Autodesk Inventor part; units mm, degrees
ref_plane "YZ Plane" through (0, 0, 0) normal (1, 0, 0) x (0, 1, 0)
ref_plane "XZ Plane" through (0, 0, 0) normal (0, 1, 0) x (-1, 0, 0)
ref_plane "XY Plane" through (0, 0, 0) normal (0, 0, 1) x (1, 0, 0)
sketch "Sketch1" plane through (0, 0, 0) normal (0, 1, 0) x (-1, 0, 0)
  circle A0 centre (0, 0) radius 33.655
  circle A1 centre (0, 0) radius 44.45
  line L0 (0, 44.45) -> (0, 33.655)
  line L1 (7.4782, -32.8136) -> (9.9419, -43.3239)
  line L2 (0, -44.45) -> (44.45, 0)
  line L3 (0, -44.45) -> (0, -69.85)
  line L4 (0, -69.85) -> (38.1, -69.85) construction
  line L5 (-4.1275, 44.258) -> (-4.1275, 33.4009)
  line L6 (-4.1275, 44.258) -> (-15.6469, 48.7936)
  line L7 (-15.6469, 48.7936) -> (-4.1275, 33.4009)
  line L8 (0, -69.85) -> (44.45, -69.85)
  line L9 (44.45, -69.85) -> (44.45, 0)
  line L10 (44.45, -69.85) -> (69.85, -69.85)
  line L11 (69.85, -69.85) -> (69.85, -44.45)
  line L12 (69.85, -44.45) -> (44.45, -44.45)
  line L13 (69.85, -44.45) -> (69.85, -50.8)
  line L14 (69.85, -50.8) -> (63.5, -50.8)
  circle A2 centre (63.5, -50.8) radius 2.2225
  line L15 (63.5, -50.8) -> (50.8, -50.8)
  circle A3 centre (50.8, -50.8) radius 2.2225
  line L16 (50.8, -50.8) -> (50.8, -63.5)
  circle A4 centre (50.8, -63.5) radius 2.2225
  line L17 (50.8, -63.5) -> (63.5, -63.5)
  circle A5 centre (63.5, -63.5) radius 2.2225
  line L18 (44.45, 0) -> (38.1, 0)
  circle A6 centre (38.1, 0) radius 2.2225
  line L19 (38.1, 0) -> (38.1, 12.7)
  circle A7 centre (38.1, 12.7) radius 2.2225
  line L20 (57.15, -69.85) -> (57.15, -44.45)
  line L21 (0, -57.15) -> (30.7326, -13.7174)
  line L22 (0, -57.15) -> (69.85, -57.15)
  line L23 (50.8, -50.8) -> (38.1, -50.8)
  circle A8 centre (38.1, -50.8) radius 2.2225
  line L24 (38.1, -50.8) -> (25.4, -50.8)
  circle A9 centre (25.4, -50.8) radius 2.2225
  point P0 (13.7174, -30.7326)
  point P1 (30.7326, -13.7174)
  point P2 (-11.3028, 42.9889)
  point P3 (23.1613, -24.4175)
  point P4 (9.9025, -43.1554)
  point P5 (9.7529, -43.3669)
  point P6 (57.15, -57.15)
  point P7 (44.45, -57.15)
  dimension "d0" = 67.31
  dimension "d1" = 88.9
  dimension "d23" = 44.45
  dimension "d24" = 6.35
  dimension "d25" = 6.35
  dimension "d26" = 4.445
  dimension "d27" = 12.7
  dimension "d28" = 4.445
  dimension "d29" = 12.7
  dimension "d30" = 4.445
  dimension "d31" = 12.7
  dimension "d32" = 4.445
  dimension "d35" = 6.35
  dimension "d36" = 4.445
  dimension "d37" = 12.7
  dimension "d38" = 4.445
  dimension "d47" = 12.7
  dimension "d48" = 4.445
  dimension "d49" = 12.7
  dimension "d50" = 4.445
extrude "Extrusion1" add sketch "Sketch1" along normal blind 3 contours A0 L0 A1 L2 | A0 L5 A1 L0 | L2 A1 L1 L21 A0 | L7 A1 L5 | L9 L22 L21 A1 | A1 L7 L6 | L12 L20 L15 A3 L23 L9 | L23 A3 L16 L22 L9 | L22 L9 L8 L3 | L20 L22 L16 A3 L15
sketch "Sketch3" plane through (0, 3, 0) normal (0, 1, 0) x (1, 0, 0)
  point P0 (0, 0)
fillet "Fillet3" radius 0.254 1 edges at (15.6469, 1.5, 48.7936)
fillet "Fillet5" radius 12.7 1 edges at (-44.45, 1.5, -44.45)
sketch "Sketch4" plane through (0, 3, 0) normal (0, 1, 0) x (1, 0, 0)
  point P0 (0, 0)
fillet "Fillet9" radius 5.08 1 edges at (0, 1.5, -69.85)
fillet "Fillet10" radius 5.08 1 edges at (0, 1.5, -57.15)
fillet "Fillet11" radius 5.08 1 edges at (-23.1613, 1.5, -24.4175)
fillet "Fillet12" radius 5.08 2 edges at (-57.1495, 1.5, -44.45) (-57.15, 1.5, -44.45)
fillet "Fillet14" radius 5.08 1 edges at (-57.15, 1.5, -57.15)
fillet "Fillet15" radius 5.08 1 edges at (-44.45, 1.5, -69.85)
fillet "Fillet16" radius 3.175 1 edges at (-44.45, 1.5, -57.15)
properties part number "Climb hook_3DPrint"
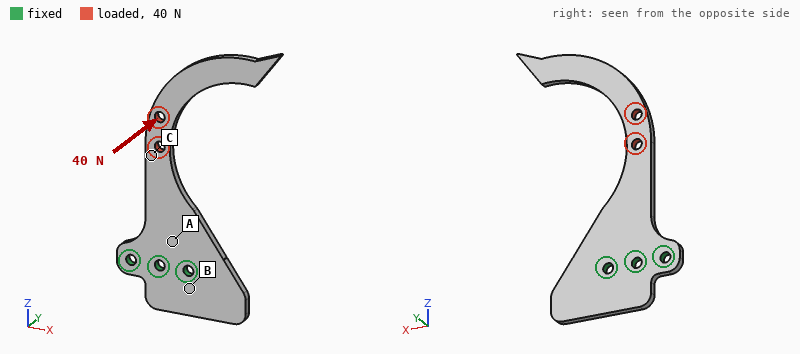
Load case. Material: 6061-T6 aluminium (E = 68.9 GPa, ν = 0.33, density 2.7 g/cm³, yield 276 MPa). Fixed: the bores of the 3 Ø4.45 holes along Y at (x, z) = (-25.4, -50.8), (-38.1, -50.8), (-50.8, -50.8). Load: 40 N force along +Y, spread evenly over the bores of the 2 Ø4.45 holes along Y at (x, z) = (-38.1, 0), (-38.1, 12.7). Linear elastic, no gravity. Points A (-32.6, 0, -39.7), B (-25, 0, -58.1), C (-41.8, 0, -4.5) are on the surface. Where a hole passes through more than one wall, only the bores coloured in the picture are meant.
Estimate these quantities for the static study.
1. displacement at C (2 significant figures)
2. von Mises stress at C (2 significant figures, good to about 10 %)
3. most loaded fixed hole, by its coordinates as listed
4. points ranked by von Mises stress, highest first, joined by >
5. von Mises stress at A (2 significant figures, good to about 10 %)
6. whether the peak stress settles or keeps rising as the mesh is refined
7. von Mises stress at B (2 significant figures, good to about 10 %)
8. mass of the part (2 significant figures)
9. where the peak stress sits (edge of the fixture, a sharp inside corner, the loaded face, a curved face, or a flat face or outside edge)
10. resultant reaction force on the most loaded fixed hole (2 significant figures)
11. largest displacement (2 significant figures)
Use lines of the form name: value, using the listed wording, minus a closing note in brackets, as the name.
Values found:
displacement at C: 0.41 mm
von Mises stress at C: 28 MPa
most loaded fixed hole, by its coordinates as listed: (-38.1, -50.8)
points ranked by von Mises stress, highest first, joined by >: A > C > B
von Mises stress at A: 36 MPa
whether the peak stress settles or keeps rising as the mesh is refined: keeps rising
von Mises stress at B: 5.7 MPa
mass of the part: 23 g
where the peak stress sits: edge of the fixture
resultant reaction force on the most loaded fixed hole: 40 N
largest displacement: 1.4 mm
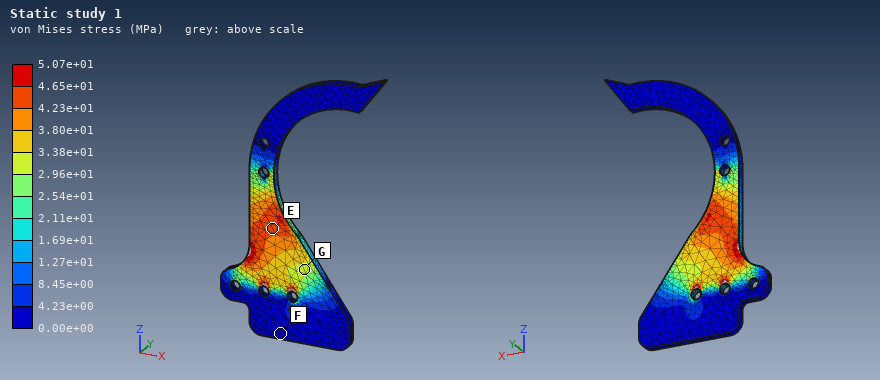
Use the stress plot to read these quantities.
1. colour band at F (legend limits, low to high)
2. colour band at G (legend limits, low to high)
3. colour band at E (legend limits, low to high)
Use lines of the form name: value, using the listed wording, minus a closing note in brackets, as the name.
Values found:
colour band at F: 0.00e+00 to 4.23e+00 MPa
colour band at G: 2.96e+01 to 3.38e+01 MPa
colour band at E: 4.23e+01 to 4.65e+01 MPa
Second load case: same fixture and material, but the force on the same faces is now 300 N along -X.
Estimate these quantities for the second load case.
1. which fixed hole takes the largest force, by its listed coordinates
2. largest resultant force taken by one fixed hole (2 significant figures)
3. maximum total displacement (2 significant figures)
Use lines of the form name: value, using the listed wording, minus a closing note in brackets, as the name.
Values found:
which fixed hole takes the largest force, by its listed coordinates: (-25.4, -50.8)
largest resultant force taken by one fixed hole: 820 N
maximum total displacement: 0.41 mm
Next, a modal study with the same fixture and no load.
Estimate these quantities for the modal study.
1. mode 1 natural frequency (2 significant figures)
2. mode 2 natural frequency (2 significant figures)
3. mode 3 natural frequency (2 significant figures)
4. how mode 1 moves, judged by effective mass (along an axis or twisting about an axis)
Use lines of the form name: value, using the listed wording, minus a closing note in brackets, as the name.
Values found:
mode 1 natural frequency: 250 Hz
mode 2 natural frequency: 920 Hz
mode 3 natural frequency: 1200 Hz
how mode 1 moves, judged by effective mass: along Y
